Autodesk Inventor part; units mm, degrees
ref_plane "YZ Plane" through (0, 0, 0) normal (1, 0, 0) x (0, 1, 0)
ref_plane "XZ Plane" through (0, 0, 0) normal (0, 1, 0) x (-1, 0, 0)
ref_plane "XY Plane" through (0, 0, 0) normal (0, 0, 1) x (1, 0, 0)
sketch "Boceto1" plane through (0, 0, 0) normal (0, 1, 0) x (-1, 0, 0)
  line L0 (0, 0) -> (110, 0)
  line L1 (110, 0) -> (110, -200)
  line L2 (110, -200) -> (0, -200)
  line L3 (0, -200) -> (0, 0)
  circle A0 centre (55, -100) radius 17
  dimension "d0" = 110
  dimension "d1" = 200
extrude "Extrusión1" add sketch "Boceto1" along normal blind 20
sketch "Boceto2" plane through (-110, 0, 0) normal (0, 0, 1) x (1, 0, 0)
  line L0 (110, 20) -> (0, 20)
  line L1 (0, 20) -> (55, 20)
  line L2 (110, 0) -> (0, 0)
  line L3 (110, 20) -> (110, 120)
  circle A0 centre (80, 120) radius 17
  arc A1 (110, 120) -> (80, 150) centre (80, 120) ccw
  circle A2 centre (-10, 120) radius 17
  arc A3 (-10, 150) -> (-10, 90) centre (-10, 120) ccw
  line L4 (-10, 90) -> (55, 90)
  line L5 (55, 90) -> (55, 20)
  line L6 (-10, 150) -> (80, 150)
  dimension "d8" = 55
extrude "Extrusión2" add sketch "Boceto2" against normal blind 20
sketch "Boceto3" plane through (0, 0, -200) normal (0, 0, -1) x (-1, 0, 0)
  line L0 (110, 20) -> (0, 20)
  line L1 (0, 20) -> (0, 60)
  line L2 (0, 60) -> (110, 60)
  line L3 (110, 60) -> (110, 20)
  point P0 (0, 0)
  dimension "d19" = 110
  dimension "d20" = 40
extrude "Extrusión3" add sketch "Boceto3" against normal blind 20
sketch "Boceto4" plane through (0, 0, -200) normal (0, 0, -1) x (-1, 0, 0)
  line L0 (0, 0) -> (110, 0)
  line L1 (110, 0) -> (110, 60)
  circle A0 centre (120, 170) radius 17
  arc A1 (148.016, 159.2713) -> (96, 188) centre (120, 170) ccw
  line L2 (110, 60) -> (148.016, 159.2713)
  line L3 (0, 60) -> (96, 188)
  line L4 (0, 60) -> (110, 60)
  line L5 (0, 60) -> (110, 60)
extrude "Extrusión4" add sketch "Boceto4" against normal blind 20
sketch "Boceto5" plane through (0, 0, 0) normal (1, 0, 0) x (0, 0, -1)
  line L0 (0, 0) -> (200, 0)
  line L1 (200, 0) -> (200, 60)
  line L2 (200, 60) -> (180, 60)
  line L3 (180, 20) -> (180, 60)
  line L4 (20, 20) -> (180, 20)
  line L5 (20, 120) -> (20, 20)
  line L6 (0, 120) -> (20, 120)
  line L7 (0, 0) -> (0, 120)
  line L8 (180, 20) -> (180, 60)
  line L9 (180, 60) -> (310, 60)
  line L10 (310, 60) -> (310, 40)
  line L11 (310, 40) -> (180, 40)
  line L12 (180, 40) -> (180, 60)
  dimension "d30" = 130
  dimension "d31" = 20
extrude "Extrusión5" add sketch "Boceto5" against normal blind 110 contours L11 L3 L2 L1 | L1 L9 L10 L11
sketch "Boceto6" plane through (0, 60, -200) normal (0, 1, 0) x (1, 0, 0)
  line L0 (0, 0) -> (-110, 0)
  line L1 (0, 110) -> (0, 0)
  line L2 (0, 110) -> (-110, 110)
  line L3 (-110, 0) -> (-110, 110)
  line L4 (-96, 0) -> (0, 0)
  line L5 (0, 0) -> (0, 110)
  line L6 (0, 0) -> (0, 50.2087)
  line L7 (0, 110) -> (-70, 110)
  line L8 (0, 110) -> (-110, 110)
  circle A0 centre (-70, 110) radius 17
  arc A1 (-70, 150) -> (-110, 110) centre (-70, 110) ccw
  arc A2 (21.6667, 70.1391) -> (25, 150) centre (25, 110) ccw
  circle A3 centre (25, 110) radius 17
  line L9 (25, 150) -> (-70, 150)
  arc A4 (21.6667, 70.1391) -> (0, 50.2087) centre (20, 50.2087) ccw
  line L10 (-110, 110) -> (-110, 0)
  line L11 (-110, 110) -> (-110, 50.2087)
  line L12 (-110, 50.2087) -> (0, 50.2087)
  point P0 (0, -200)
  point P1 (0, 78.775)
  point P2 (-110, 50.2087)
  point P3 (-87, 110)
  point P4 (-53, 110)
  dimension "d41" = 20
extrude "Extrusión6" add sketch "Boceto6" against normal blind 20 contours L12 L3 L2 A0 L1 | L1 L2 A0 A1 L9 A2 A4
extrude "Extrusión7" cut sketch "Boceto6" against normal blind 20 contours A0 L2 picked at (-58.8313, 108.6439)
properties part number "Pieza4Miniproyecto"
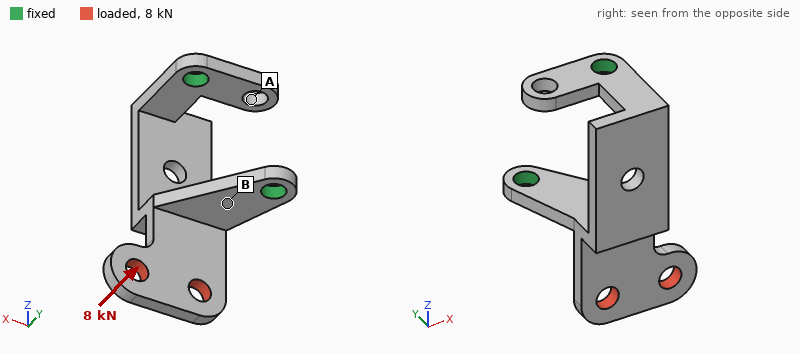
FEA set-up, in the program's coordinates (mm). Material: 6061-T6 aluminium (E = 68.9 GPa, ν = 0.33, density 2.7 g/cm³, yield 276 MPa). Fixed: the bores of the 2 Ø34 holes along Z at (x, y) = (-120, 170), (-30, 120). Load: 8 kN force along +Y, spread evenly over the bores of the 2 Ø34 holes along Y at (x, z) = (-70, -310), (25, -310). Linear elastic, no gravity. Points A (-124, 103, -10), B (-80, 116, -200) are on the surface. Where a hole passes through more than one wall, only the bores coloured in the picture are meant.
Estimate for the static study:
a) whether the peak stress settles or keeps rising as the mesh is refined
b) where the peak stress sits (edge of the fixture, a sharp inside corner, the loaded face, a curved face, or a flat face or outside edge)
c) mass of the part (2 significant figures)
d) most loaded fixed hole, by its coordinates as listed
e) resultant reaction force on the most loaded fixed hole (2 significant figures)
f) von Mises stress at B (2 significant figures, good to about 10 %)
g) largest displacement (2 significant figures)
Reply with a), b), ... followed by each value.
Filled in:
a) keeps rising
b) edge of the fixture
c) 3.5 kg
d) (-120, 170)
e) 12 kN
f) 59 MPa
g) 2.8 mm
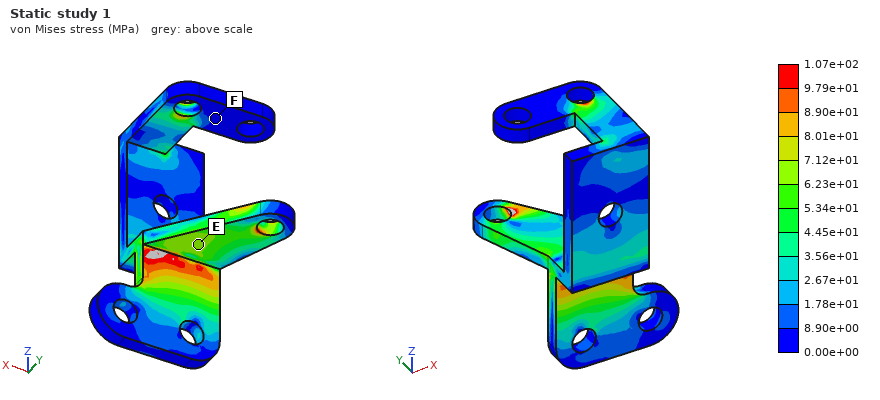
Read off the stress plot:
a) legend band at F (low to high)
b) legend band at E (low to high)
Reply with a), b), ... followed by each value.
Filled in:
a) 0.00e+00 to 8.90e+00 MPa
b) 6.23e+01 to 7.12e+01 MPa
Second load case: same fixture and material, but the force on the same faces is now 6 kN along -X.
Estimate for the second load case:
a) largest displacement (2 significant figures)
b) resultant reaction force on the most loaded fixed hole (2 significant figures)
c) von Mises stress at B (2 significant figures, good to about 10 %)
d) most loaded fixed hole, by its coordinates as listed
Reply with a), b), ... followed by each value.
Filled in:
a) 0.96 mm
b) 8.5 kN
c) 43 MPa
d) (-120, 170)
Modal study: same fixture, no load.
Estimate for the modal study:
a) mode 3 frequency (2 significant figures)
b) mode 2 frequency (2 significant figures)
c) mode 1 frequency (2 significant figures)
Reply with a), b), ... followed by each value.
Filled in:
a) 670 Hz
b) 530 Hz
c) 370 Hz
